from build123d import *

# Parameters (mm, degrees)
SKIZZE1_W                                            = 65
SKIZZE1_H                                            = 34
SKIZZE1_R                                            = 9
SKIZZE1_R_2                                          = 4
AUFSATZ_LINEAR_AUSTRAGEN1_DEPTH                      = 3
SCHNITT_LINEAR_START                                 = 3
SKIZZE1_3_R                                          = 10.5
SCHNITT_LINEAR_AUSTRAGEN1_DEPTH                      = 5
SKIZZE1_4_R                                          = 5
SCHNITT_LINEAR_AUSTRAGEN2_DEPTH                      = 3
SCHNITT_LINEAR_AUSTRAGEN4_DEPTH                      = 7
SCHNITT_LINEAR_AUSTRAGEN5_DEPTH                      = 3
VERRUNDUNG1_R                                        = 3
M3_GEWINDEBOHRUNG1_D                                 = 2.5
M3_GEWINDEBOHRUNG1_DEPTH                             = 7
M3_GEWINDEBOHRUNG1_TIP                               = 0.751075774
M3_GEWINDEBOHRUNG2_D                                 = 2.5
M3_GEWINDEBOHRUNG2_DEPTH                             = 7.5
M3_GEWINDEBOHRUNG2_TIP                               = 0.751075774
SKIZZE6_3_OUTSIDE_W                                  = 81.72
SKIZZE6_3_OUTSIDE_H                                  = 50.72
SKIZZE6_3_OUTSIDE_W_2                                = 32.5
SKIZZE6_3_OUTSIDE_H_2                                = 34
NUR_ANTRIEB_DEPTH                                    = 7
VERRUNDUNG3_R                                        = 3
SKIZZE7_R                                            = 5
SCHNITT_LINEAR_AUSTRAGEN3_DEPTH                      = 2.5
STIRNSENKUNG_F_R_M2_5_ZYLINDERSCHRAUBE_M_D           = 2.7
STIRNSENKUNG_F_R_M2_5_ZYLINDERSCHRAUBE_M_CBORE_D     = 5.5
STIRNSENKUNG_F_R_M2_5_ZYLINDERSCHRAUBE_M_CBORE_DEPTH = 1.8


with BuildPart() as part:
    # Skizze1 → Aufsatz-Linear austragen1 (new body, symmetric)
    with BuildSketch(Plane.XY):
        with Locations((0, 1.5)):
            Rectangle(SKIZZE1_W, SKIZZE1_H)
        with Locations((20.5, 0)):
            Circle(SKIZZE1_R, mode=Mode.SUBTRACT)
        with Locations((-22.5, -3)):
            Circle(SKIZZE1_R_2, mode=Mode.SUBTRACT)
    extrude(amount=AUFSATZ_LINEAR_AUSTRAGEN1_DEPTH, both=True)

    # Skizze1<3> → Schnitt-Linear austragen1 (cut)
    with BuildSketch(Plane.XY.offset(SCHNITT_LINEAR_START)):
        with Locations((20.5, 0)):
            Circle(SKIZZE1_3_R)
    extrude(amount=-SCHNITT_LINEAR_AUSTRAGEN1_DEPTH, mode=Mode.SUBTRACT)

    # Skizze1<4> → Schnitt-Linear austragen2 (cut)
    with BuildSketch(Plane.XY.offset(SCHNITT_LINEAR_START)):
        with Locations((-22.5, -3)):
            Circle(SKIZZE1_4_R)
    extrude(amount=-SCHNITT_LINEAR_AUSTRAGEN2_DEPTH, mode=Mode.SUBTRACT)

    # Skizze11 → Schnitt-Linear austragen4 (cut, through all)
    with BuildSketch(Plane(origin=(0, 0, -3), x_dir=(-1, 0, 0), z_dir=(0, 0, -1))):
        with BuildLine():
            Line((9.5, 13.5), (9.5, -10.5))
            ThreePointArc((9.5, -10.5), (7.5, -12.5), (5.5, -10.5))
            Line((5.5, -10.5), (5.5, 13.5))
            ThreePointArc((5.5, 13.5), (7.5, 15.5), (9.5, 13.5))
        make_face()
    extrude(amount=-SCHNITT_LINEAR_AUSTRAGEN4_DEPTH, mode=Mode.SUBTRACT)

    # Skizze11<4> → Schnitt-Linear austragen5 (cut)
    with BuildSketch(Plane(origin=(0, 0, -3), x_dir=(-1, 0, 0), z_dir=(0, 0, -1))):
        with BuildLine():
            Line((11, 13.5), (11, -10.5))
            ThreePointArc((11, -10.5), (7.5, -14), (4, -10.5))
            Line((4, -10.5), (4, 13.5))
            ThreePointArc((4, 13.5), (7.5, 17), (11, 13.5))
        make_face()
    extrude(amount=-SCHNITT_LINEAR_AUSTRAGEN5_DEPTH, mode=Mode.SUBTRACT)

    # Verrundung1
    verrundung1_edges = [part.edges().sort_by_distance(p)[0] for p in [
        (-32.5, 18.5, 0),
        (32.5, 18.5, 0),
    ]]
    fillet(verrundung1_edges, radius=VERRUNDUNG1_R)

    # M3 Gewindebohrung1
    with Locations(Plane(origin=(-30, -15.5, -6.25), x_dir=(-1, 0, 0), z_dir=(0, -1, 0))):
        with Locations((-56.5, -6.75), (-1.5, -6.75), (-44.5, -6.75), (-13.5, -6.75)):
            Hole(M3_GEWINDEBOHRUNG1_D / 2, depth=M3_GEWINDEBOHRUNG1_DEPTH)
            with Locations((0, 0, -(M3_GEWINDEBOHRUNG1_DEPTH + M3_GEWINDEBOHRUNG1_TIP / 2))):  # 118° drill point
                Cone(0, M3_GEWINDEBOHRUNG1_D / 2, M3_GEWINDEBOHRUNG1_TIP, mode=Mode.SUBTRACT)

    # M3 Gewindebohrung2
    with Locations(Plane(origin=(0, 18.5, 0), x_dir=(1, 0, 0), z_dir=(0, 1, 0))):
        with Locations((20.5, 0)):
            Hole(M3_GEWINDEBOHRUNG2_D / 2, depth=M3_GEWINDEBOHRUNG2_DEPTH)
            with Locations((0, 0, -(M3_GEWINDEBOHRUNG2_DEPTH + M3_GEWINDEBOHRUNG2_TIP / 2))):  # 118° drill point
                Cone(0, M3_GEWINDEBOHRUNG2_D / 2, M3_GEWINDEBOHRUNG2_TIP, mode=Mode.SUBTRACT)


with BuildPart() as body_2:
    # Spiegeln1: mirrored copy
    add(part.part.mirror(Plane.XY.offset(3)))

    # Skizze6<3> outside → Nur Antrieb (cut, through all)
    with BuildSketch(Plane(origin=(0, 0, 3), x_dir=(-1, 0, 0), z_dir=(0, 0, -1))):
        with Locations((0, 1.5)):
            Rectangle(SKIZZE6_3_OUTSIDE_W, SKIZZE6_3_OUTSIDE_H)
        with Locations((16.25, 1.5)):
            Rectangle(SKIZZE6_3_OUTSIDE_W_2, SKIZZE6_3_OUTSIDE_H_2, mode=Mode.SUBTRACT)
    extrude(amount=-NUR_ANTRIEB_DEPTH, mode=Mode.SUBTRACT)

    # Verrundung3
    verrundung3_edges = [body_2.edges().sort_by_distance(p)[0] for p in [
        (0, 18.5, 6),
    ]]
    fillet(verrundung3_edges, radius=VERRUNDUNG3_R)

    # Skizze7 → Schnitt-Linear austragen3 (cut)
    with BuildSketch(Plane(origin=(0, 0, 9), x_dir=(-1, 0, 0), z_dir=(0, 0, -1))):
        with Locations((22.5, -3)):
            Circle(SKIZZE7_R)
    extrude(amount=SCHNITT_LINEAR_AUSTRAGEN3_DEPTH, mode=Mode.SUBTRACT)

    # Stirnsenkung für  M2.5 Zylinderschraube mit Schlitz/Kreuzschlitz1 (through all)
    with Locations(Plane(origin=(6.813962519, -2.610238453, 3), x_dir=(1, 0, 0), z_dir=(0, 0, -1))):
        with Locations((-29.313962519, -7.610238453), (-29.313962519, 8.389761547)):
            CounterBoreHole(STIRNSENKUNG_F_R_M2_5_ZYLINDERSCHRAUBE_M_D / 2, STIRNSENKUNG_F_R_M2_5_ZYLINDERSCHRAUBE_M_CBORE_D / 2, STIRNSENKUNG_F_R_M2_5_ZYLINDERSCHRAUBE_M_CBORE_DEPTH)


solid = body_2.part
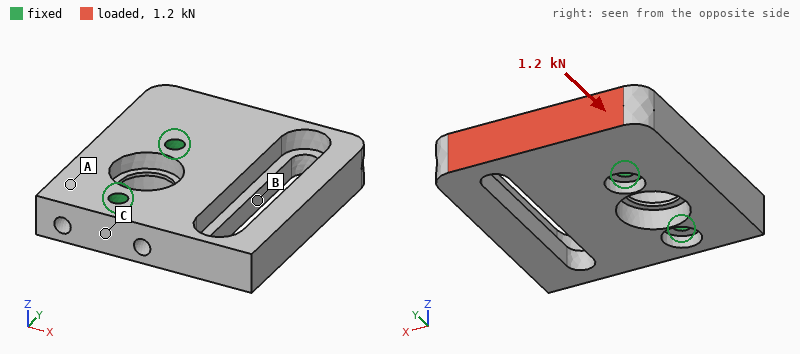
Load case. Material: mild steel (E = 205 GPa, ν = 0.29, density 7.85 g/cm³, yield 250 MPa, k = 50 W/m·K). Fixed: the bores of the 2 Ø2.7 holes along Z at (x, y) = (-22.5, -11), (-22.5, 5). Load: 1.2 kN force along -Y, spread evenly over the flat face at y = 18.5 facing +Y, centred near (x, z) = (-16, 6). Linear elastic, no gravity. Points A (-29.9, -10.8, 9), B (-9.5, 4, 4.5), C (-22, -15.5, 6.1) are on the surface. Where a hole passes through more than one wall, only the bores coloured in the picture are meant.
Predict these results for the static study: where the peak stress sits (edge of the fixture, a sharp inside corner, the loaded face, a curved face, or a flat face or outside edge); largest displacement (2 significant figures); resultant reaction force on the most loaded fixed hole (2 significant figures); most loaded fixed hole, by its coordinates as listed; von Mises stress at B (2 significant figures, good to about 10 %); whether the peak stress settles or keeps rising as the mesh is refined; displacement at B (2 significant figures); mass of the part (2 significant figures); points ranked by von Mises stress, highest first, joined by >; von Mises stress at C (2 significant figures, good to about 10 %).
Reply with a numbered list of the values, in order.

1. edge of the fixture
2. 6.6 µm
3. 970 N
4. (-22.5, 5)
5. 22 MPa
6. keeps rising
7. 2.0 µm
8. 39 g
9. B > C > A
10. 11 MPa
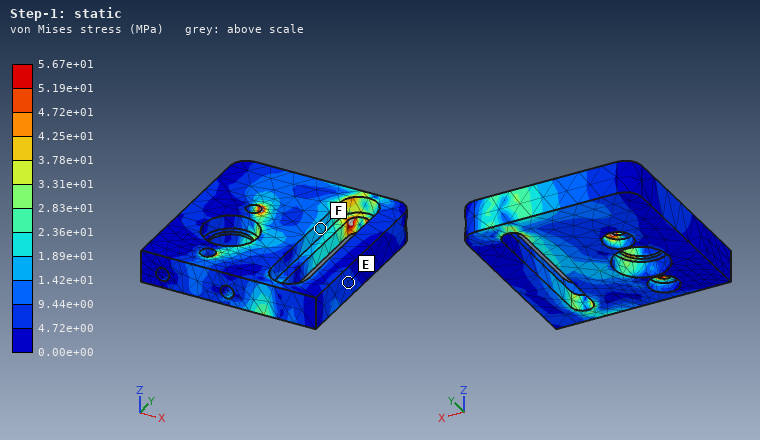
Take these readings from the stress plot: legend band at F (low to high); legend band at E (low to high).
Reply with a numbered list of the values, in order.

1. 1.42e+01 to 1.89e+01 MPa
2. 4.72e+00 to 9.44e+00 MPa
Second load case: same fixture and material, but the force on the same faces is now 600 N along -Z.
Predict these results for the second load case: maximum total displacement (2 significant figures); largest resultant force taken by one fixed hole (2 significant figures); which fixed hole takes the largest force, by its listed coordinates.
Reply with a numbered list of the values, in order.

1. 32 µm
2. 870 N
3. (-22.5, 5)
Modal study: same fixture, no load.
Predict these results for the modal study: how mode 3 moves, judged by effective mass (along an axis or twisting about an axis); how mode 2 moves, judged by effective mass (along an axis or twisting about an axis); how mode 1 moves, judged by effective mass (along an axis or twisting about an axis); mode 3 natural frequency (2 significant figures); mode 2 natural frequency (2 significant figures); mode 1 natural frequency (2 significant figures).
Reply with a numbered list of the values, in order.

1. along Y
2. twisting about X
3. along Z
4. 12 kHz
5. 10 kHz
6. 5500 Hz
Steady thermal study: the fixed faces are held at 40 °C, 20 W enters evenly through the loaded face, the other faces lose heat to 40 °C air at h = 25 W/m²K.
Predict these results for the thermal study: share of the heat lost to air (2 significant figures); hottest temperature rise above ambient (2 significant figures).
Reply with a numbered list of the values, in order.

1. 9.1 %
2. 69 K
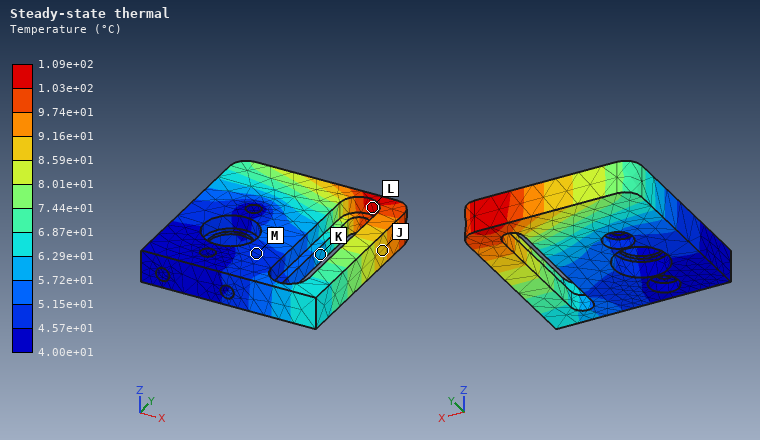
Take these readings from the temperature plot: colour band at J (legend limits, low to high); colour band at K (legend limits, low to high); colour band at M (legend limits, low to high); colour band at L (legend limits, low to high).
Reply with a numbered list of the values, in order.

1. 8.59e+01 to 9.16e+01 °C
2. 5.72e+01 to 6.29e+01 °C
3. 4.57e+01 to 5.15e+01 °C
4. 1.03e+02 to 1.09e+02 °C
